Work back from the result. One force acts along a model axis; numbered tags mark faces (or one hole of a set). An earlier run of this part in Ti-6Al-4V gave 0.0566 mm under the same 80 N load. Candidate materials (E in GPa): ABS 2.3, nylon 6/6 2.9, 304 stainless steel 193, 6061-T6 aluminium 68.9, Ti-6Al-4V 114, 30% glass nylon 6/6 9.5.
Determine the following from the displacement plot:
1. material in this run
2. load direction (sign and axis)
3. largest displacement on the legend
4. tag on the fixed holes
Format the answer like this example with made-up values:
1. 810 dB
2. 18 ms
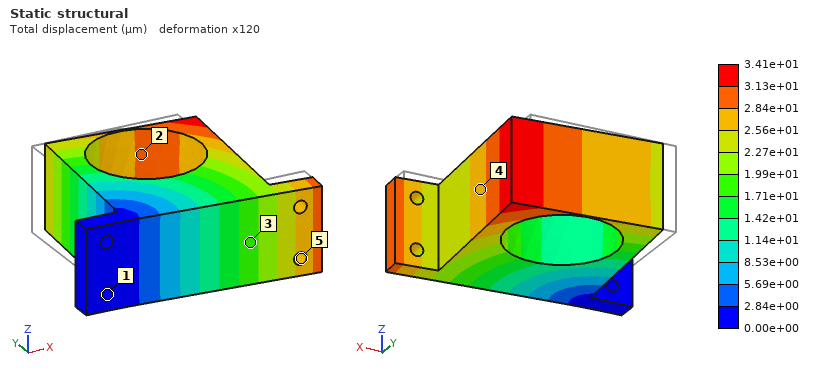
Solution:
1. 304 stainless steel
2. -Y
3. 3.41e+01 µm
4. 1
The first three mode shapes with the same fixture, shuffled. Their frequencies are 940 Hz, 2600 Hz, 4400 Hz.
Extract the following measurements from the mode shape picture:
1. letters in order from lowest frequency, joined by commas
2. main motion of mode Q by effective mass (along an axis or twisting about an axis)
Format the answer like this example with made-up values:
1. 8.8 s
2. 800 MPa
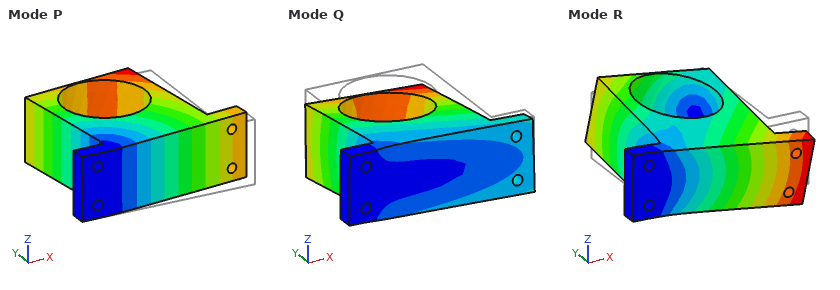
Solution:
1. P, Q, R
2. along Z
